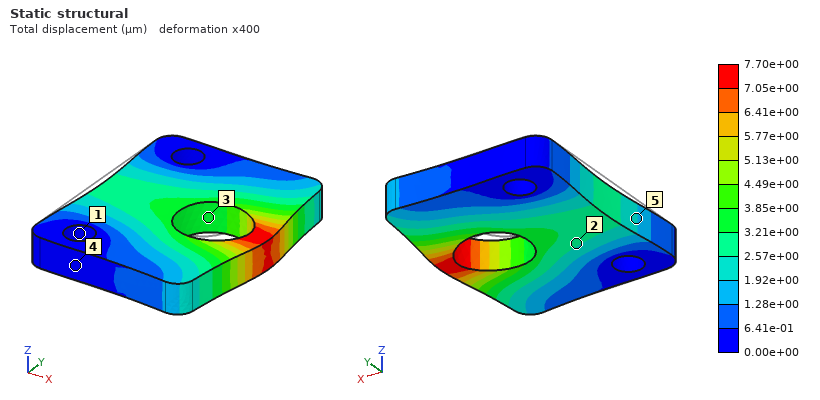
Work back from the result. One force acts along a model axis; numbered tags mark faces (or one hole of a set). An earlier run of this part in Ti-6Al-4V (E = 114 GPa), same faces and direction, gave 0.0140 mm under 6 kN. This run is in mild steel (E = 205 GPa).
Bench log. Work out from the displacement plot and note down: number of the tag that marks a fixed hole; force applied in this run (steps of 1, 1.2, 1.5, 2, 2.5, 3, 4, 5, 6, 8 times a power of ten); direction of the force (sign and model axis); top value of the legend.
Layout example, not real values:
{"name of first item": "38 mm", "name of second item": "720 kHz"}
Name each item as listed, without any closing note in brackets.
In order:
{"number of the tag that marks a fixed hole": "1", "force applied in this run": "6 kN", "direction of the force": "+X", "top value of the legend": "7.70e+00 µm"}
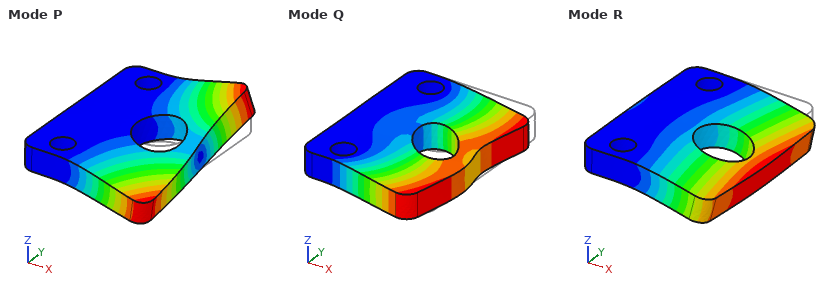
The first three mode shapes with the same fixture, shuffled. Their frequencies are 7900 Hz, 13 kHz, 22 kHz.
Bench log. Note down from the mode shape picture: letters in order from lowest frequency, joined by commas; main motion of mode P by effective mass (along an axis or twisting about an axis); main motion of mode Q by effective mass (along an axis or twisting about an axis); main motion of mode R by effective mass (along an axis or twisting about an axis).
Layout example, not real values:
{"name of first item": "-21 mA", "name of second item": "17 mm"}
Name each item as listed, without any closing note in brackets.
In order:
{"letters in order from lowest frequency, joined by commas": "R, P, Q", "main motion of mode P by effective mass": "twisting about X", "main motion of mode Q by effective mass": "along Y", "main motion of mode R by effective mass": "along Z"}
